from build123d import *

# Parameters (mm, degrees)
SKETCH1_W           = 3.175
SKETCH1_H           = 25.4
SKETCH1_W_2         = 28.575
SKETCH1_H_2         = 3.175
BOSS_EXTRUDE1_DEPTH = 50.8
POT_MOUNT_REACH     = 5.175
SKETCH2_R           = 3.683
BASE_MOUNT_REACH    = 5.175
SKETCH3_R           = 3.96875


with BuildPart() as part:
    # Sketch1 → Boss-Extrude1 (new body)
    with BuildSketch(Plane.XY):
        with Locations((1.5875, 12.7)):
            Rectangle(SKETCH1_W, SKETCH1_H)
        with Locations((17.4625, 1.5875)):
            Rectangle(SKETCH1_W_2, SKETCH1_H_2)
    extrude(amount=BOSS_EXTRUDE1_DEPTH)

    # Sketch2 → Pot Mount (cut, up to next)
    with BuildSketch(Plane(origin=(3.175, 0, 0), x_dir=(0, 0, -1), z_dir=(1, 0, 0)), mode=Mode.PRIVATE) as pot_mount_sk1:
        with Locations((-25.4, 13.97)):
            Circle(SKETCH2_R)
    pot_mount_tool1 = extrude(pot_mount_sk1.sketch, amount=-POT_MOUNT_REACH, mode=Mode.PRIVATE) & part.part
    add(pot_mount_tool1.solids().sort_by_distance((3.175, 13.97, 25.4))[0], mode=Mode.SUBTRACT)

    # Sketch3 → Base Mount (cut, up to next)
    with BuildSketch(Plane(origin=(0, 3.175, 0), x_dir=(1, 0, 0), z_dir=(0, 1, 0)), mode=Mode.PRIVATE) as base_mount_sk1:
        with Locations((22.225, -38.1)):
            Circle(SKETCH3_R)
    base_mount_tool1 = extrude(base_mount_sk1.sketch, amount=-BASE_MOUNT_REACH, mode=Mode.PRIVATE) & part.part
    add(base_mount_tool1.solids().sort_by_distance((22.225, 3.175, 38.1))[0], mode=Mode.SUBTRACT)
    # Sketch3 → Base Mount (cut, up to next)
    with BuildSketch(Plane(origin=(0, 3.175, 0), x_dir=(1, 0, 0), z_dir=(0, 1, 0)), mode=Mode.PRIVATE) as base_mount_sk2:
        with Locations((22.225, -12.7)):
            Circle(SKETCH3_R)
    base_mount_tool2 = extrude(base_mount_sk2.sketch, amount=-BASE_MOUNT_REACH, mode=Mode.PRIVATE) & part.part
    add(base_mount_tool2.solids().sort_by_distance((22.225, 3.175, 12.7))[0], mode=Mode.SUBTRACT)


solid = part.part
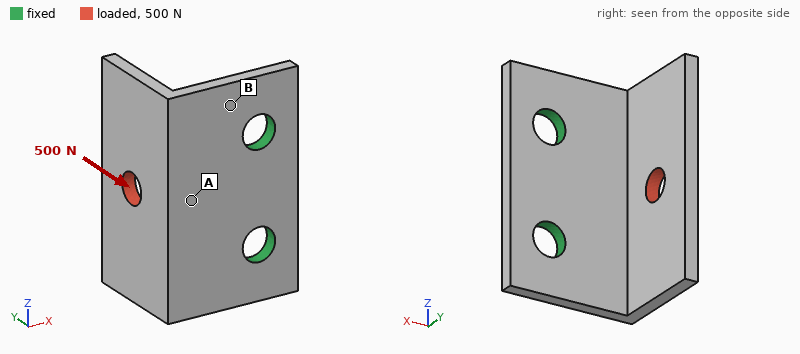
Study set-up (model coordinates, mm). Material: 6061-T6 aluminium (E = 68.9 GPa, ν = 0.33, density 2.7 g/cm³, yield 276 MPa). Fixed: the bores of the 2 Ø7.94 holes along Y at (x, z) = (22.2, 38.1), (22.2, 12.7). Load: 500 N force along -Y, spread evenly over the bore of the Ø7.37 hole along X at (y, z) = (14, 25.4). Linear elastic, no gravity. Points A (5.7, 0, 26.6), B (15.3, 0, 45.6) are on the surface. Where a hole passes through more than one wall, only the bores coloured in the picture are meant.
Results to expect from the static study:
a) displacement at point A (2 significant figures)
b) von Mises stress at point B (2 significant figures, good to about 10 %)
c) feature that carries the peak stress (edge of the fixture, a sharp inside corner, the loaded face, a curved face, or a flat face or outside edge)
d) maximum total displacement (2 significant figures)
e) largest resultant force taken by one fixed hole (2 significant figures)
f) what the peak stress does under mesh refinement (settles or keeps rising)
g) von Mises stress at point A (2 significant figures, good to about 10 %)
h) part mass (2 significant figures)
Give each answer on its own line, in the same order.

0.076 mm
65 MPa
edge of the fixture
0.24 mm
250 N
keeps rising
24 MPa
22 g
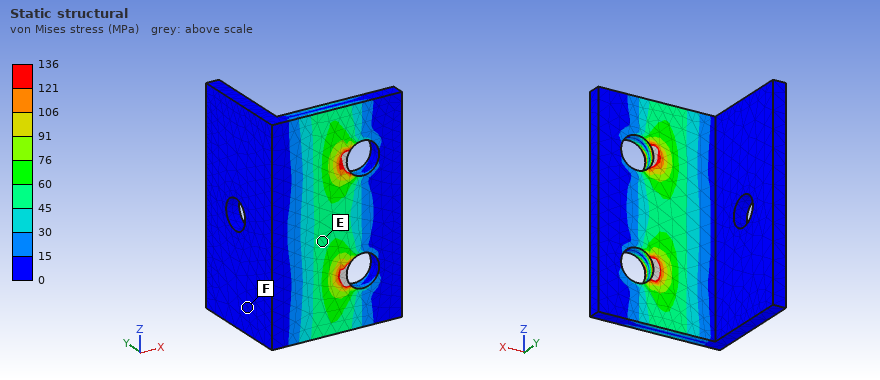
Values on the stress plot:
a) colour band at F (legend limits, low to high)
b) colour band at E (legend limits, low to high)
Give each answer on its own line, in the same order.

0 to 15 MPa
45 to 60 MPa
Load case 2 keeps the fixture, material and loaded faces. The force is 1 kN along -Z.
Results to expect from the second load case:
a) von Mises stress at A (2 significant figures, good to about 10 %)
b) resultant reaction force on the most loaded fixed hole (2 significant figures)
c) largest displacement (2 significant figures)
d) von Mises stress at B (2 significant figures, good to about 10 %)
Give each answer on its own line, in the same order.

35 MPa
860 N
0.21 mm
65 MPa
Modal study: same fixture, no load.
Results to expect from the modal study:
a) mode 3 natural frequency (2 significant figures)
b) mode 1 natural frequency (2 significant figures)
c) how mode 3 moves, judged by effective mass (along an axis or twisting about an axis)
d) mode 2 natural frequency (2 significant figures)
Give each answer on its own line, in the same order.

5500 Hz
2000 Hz
along Y
3300 Hz
